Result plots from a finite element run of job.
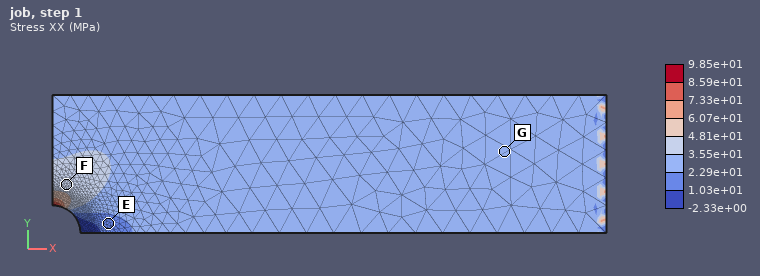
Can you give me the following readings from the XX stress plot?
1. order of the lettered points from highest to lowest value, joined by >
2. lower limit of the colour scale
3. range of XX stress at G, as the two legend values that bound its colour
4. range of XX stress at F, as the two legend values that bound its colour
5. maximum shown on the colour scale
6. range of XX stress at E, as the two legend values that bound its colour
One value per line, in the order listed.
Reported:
F > G > E
-2.33e+00 MPa
2.29e+01 to 3.55e+01 MPa
3.55e+01 to 4.81e+01 MPa
9.85e+01 MPa
1.03e+01 to 2.29e+01 MPa
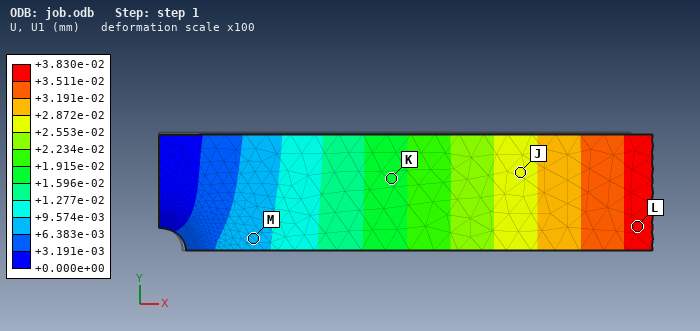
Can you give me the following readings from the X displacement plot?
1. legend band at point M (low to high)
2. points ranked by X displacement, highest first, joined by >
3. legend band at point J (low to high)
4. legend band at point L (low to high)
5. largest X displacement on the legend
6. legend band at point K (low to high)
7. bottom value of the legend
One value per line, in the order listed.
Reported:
+6.383e-03 to +9.574e-03 mm
L > J > K > M
+2.553e-02 to +2.872e-02 mm
+3.511e-02 to +3.830e-02 mm
+3.830e-02 mm
+1.596e-02 to +1.915e-02 mm
+0.000e+00 mm
